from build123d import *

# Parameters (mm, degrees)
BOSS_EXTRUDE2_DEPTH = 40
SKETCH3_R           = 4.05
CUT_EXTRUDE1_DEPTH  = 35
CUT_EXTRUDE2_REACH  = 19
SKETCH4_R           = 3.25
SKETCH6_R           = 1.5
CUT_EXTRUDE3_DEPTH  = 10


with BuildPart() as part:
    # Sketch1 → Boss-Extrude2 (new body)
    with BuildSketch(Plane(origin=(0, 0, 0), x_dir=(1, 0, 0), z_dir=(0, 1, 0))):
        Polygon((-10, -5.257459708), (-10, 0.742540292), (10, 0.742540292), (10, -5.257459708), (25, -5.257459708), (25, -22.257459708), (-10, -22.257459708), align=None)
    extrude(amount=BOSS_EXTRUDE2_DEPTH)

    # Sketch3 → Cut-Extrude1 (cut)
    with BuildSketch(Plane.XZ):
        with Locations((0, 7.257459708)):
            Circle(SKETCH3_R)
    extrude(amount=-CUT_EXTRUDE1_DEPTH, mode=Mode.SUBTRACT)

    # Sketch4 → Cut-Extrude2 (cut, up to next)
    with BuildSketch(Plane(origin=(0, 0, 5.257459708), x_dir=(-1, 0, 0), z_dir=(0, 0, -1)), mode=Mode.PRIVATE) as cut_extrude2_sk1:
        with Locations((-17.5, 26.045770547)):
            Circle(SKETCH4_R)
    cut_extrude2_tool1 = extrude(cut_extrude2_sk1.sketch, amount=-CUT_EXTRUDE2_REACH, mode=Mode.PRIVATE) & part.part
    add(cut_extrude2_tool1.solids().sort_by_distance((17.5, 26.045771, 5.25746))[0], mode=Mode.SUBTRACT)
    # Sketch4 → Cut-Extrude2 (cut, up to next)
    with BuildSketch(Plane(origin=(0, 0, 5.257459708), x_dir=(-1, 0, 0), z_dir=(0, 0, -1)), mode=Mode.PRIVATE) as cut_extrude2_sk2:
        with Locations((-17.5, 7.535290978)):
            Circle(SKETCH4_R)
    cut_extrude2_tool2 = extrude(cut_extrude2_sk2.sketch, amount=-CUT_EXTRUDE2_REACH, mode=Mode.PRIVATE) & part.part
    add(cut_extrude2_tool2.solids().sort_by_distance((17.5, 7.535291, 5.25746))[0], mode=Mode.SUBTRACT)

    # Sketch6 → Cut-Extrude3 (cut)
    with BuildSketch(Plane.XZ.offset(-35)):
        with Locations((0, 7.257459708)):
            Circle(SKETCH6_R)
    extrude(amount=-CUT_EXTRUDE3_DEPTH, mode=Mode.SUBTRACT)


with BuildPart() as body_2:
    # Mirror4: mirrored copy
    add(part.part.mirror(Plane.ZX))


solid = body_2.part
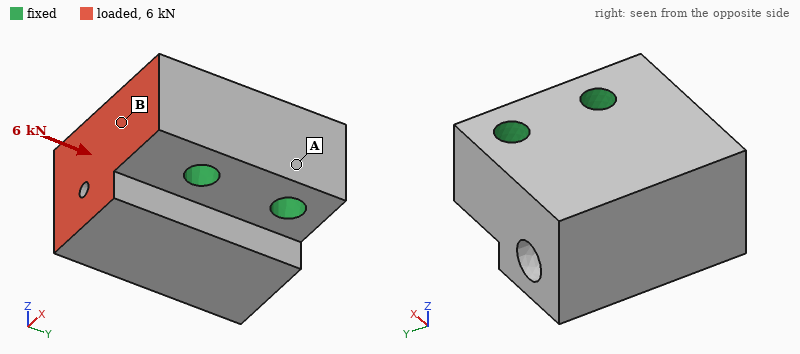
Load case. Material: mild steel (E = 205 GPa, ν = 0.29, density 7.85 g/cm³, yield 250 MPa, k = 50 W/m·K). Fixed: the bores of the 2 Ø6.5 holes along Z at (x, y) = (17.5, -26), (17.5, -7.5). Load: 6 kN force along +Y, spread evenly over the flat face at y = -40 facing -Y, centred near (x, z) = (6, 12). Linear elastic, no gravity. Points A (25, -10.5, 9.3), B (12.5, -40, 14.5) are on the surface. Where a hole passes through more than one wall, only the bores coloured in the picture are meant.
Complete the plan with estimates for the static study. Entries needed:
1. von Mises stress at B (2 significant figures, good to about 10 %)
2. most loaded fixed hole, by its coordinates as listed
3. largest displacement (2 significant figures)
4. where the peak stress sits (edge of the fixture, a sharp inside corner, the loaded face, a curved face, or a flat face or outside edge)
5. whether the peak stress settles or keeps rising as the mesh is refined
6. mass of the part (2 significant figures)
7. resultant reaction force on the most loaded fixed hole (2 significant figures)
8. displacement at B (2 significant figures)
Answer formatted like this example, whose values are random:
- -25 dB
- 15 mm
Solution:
- 13 MPa
- (17.5, -26)
- 4.5 µm
- edge of the fixture
- keeps rising
- 200 g
- 4.9 kN
- 2.0 µm
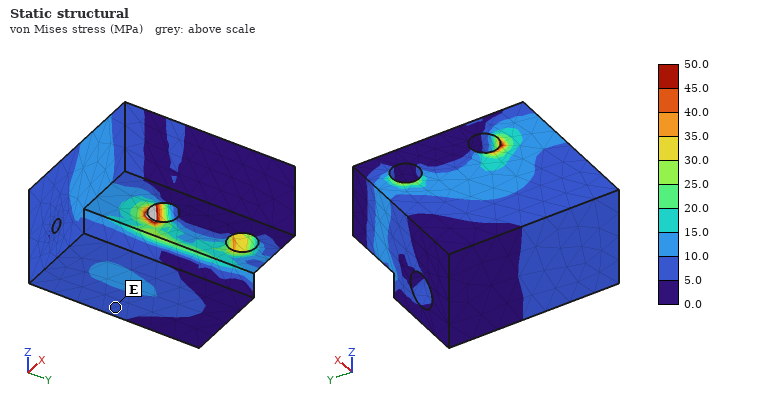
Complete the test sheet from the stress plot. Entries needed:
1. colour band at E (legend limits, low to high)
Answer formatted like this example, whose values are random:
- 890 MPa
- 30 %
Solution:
- 5.0 to 10.0 MPa
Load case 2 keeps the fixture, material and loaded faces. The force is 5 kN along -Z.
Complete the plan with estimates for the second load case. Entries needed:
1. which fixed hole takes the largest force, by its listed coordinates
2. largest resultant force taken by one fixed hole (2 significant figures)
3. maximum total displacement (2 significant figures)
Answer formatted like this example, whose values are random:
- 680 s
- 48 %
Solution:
- (17.5, -26)
- 5.6 kN
- 12 µm
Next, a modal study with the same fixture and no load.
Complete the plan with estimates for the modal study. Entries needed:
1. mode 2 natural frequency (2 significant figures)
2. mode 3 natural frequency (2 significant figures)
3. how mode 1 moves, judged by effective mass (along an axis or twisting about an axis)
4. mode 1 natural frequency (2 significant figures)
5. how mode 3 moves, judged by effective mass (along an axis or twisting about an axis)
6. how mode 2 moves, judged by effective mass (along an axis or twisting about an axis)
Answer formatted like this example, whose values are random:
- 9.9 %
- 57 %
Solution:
- 17 kHz
- 20 kHz
- along Z
- 13 kHz
- twisting about X
- along Y
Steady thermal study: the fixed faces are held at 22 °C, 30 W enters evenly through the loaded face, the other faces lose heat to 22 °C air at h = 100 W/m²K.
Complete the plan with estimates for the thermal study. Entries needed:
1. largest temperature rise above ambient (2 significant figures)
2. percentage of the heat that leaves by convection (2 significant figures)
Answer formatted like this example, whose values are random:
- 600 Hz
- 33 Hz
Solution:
- 21 K
- 13 %
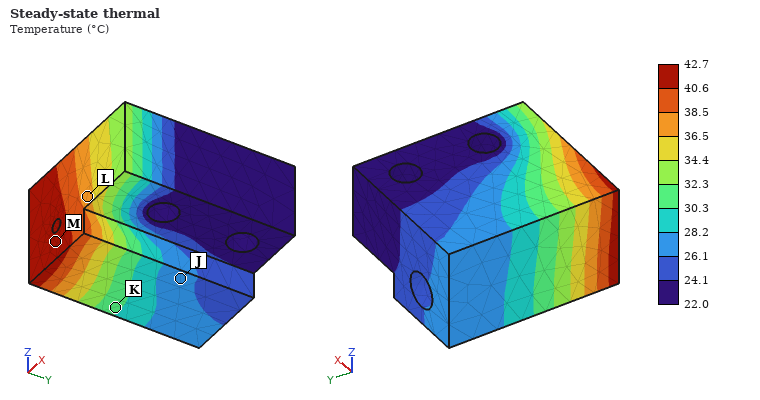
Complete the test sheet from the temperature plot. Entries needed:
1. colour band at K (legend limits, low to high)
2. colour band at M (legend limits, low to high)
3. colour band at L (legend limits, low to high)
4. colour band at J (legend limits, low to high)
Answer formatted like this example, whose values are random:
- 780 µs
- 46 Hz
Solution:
- 30.3 to 32.3 °C
- 40.6 to 42.7 °C
- 36.5 to 38.5 °C
- 26.1 to 28.2 °C
